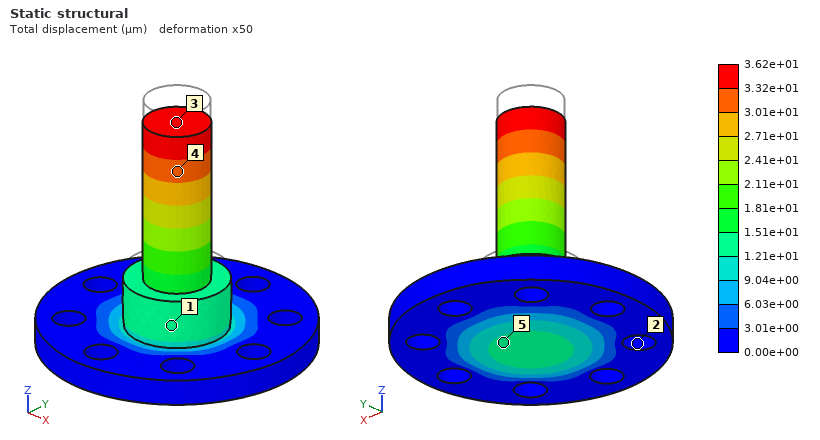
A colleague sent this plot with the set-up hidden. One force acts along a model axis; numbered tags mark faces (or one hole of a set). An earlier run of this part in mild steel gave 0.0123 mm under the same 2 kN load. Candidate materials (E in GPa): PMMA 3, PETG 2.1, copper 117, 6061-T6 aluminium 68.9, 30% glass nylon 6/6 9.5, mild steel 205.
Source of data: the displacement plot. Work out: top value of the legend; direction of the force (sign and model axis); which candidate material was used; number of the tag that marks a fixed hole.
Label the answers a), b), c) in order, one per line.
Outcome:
a) 3.62e+01 µm
b) -Z
c) 6061-T6 aluminium
d) 2
